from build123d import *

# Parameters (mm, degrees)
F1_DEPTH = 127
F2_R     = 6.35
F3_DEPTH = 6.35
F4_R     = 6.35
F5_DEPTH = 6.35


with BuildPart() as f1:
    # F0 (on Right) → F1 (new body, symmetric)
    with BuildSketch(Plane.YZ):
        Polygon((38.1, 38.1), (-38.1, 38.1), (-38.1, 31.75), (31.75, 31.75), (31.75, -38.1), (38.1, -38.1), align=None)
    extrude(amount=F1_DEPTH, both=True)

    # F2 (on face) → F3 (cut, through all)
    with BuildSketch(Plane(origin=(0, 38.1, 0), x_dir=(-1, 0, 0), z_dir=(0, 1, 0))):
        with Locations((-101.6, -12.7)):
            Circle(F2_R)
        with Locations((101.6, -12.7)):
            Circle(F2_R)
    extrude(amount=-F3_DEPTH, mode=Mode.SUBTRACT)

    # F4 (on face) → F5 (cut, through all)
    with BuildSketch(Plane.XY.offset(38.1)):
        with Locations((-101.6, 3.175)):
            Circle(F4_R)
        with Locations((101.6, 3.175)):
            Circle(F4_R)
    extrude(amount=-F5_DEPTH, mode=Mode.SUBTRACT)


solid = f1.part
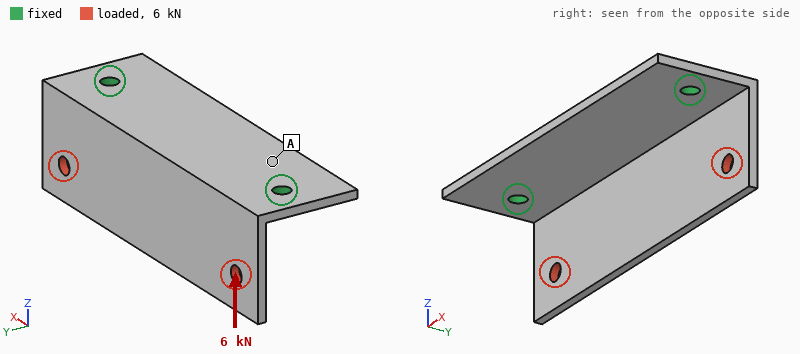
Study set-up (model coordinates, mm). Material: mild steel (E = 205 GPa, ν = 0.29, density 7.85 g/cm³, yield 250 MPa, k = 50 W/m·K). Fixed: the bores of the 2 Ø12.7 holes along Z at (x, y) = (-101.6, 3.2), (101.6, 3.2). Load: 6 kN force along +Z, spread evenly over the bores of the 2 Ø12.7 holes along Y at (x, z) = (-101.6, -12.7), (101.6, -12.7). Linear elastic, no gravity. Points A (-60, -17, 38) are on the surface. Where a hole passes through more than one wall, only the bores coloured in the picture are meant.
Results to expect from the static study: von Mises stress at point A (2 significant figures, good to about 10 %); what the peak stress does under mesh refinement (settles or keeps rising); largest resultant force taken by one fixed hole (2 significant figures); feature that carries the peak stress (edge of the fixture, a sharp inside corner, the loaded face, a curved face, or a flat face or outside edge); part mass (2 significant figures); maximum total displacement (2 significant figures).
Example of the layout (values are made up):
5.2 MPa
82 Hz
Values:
21 MPa
keeps rising
3.0 kN
edge of the fixture
1.8 kg
0.32 mm
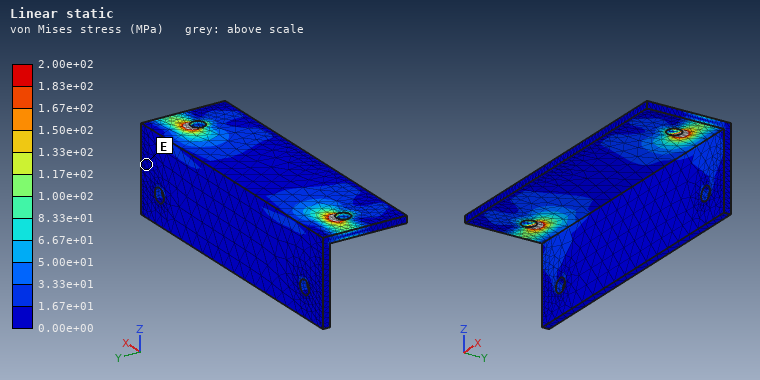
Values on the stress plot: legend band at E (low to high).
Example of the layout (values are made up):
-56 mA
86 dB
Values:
0.00e+00 to 1.67e+01 MPa
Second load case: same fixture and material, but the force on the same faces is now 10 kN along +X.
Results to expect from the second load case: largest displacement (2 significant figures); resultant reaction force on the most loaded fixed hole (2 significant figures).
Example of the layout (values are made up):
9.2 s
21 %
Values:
0.18 mm
5.7 kN
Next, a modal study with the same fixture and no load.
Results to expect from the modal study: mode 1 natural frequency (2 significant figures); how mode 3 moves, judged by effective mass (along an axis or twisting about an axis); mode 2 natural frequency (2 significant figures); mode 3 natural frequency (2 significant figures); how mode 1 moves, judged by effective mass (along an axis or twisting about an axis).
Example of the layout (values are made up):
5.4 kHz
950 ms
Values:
510 Hz
along Z
840 Hz
1100 Hz
along Y
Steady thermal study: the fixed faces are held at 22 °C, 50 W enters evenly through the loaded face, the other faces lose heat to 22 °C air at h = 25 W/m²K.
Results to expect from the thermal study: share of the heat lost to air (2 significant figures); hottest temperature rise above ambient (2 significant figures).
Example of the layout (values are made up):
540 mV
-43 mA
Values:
63 %
59 K
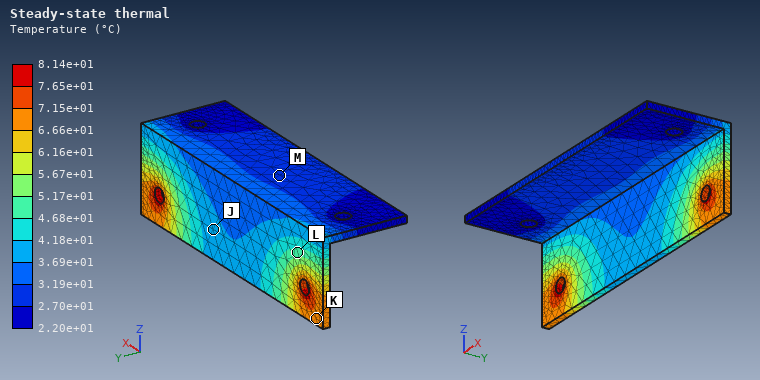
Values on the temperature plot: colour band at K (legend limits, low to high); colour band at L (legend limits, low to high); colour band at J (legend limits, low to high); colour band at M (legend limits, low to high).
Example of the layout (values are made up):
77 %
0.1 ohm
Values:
6.66e+01 to 7.15e+01 °C
4.68e+01 to 5.17e+01 °C
3.69e+01 to 4.18e+01 °C
2.70e+01 to 3.19e+01 °C
